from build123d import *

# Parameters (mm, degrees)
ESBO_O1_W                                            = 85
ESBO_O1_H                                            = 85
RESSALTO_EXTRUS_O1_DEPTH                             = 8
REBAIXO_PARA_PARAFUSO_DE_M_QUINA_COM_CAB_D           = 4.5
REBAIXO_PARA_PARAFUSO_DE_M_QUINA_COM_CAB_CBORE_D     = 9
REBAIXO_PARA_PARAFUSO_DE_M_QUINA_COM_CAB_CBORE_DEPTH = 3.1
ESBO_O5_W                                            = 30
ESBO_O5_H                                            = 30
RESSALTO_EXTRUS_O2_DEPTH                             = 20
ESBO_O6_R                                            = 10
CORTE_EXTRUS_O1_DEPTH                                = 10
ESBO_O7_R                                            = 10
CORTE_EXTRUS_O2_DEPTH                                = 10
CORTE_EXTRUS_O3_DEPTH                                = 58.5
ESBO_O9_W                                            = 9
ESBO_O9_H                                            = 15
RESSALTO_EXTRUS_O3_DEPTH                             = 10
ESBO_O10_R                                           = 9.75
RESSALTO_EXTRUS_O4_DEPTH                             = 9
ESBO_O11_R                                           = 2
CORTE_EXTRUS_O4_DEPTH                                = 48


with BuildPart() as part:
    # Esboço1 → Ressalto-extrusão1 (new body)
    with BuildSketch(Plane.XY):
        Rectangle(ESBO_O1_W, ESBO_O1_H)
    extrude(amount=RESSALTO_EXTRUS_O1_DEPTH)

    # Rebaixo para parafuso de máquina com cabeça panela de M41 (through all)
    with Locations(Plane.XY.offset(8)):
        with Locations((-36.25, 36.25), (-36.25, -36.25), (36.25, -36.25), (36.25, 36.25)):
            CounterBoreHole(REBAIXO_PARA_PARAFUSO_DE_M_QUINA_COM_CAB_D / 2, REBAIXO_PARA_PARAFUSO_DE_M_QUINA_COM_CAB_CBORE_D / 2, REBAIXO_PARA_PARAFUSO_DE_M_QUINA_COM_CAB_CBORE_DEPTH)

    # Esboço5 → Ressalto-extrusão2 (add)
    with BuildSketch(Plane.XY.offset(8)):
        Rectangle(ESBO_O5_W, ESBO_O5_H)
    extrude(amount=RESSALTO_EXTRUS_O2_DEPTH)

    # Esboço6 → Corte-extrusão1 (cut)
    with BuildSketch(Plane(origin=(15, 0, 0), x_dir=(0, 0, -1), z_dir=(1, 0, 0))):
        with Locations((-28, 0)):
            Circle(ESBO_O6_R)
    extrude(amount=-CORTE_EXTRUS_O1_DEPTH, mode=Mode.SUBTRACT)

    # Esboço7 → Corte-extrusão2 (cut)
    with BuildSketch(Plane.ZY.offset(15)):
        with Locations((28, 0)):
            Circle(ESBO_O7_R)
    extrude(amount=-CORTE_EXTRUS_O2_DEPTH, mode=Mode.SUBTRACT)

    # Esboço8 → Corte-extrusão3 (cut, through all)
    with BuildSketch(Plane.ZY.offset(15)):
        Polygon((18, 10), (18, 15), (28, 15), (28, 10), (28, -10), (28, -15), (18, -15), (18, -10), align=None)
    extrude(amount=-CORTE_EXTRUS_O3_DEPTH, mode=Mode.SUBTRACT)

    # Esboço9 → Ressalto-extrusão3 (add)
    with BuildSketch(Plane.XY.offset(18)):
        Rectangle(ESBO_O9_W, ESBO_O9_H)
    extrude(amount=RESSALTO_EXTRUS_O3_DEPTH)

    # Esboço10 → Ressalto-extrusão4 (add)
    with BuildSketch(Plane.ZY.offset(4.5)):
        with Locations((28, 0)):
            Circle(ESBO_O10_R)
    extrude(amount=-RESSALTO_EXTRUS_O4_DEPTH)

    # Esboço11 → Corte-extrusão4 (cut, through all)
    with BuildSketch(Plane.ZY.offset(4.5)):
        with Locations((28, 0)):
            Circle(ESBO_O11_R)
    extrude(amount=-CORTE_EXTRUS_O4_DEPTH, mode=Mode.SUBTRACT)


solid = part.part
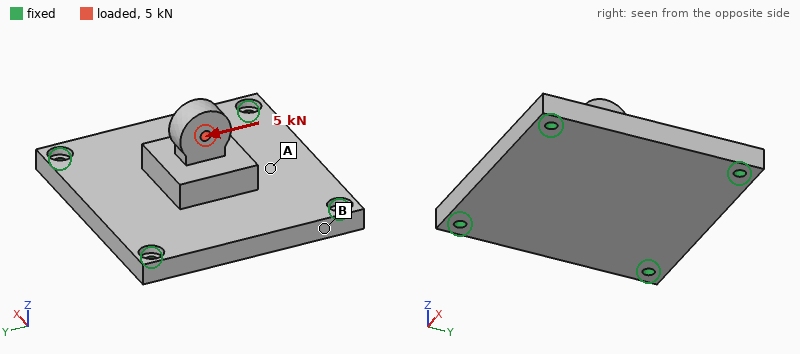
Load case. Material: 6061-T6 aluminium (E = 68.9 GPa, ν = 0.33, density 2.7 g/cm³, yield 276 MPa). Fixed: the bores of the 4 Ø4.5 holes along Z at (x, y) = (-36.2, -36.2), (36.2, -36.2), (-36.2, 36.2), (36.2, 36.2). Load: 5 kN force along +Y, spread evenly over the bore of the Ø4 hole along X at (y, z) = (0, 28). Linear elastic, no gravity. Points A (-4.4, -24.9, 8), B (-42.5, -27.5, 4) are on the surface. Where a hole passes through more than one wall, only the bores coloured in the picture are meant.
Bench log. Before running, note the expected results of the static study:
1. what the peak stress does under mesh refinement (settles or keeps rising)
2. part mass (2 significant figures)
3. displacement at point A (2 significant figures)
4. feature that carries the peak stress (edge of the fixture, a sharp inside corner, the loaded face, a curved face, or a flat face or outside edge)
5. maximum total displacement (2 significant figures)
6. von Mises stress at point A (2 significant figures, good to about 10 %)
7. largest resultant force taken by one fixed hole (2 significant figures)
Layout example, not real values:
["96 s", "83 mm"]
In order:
["keeps rising", "180 g", "0.042 mm", "edge of the fixture", "0.15 mm", "30 MPa", "1.9 kN"]
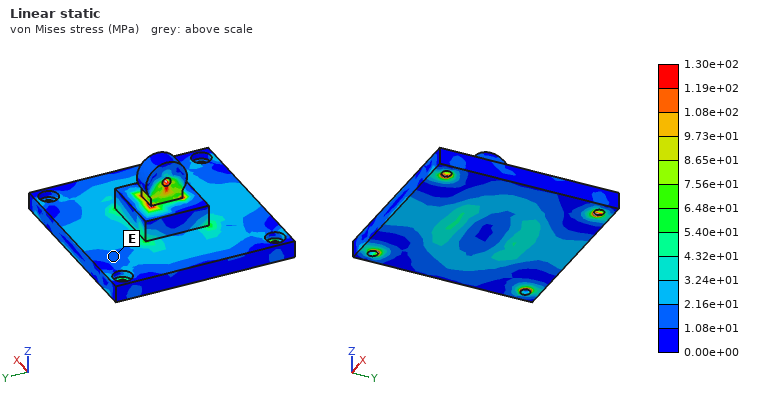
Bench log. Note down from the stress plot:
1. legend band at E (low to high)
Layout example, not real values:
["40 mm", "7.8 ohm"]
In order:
["1.08e+01 to 2.16e+01 MPa"]
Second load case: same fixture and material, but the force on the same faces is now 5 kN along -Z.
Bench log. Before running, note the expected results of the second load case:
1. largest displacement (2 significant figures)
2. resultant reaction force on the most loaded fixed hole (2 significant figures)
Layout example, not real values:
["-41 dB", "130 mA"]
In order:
["98 µm", "1.9 kN"]
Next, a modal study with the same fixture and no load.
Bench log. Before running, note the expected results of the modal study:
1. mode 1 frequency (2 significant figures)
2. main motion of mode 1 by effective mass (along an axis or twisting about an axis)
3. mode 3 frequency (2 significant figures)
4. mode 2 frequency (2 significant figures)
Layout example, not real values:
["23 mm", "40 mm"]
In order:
["3800 Hz", "along Z", "6400 Hz", "6400 Hz"]
